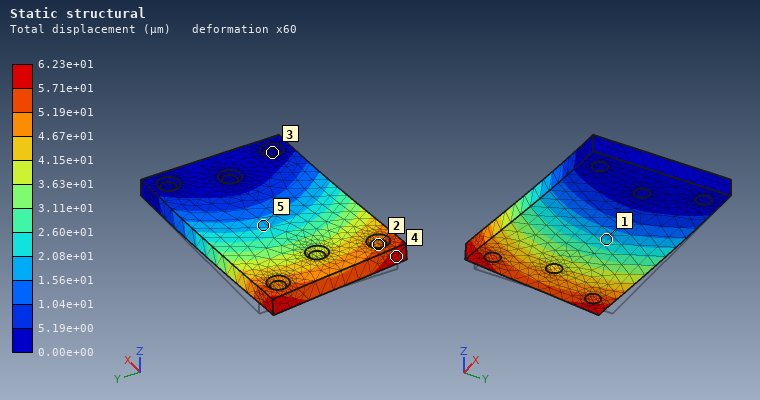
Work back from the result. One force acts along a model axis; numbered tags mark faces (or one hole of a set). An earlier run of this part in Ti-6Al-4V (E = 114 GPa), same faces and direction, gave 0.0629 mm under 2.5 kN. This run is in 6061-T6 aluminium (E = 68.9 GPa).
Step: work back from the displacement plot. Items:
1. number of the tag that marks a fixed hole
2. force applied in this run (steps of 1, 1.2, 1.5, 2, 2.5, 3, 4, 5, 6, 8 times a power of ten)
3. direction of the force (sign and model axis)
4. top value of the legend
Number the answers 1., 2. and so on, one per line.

1. 3
2. 1.5 kN
3. -Y
4. 6.23e+01 µm
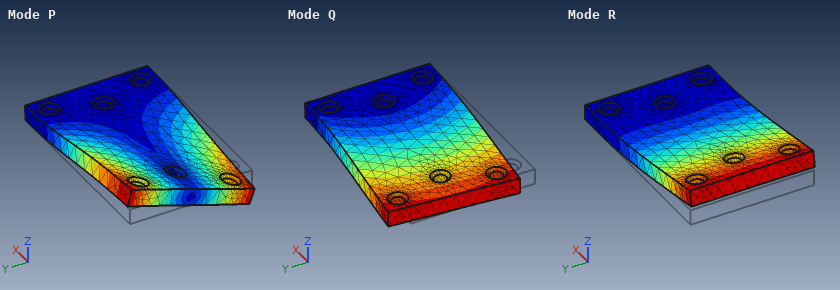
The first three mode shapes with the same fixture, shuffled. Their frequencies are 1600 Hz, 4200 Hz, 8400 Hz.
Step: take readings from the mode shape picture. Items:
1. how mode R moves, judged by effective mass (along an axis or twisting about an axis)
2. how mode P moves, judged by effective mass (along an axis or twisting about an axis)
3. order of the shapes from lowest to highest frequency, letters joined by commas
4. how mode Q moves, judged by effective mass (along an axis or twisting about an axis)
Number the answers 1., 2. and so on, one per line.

1. along Z
2. twisting about X
3. R, P, Q
4. along Y
